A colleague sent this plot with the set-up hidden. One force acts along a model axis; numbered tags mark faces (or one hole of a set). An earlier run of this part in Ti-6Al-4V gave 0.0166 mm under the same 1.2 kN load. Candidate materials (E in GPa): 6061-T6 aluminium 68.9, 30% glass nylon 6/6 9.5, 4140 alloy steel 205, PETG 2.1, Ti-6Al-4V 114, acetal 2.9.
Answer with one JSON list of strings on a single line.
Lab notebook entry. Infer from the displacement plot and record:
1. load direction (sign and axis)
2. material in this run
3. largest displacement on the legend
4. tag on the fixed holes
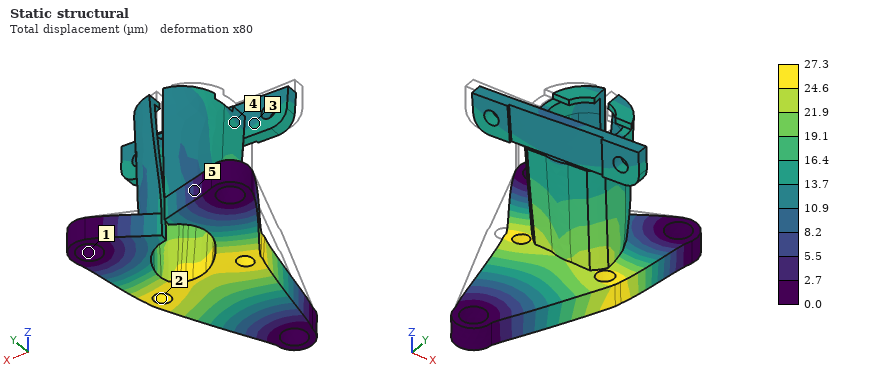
["+X", "6061-T6 aluminium", "27.3 µm", "1"]
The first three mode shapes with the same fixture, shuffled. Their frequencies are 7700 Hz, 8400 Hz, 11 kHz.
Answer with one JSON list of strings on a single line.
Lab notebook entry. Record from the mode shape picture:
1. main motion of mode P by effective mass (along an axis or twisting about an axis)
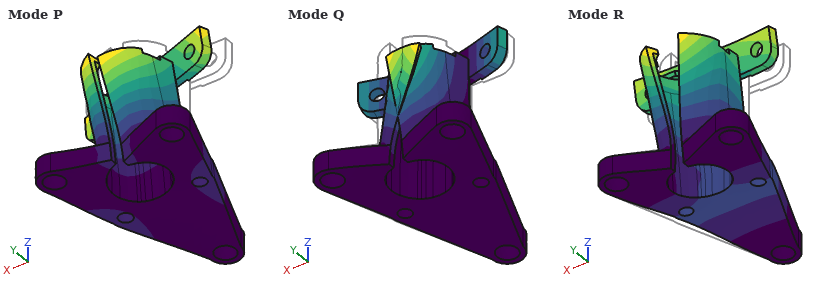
["along X"]
